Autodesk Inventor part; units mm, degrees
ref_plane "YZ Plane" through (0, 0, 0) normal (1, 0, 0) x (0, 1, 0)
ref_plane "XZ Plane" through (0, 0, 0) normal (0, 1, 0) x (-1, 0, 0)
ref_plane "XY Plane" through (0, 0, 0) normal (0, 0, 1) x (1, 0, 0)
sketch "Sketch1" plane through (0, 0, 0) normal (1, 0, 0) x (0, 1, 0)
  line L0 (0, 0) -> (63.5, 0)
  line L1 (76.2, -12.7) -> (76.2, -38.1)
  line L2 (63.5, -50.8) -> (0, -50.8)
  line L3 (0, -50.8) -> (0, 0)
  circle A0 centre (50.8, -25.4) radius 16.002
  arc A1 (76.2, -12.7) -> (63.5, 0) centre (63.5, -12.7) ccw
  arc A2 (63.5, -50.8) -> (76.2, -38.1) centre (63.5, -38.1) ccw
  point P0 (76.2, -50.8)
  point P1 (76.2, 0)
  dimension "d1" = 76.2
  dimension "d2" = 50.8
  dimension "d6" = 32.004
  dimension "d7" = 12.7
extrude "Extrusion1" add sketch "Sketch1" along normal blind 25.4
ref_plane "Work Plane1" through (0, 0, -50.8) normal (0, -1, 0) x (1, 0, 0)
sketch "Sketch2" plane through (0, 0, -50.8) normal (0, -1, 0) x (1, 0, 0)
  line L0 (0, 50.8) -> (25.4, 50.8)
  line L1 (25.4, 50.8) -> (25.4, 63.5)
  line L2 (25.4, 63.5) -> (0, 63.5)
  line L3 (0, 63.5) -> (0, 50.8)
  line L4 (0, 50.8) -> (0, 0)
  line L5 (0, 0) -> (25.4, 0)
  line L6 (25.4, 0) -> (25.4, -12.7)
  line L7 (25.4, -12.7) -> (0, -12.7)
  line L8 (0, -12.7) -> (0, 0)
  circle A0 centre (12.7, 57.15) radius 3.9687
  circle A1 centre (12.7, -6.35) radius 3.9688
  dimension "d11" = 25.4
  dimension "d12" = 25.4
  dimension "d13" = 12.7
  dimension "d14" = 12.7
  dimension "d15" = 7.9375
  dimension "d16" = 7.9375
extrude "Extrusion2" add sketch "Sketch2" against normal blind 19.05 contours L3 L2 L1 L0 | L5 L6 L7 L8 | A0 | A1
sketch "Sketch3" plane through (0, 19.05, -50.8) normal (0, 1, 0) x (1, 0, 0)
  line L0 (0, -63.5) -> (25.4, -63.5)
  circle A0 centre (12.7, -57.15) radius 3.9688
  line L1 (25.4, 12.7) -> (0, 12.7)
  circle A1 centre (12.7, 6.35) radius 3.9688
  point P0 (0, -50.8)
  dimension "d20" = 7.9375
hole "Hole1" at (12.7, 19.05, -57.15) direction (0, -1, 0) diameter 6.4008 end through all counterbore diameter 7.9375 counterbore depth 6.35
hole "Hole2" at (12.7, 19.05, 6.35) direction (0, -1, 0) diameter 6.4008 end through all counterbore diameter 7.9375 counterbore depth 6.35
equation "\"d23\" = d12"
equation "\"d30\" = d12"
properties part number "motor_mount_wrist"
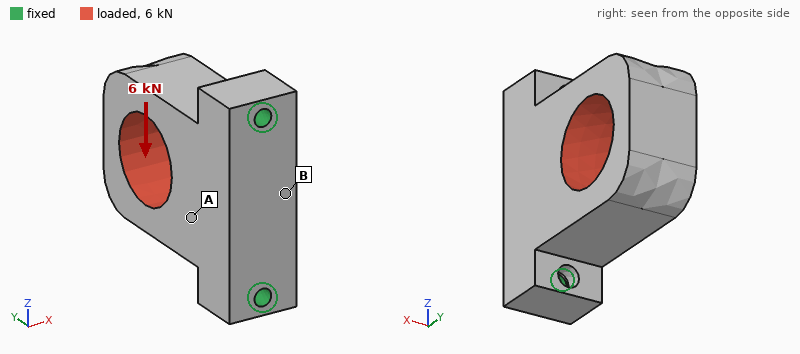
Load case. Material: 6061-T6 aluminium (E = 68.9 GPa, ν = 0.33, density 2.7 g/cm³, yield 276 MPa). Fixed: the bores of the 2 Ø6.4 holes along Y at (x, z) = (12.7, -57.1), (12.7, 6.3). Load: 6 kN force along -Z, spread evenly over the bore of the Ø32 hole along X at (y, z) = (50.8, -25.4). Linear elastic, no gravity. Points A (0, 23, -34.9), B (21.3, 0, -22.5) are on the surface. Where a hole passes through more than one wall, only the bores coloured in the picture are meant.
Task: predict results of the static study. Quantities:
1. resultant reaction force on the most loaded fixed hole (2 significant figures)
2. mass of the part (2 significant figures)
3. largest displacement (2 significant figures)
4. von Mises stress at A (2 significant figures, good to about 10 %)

5.3 kN
230 g
60 µm
13 MPa
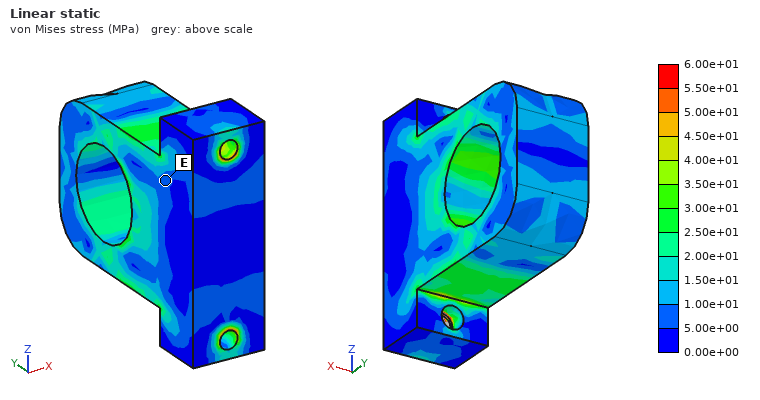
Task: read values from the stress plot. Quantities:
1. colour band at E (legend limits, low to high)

5.00e+00 to 1.00e+01 MPa
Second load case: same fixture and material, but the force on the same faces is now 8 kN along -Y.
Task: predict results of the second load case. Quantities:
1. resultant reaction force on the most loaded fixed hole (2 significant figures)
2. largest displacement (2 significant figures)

4.3 kN
19 µm
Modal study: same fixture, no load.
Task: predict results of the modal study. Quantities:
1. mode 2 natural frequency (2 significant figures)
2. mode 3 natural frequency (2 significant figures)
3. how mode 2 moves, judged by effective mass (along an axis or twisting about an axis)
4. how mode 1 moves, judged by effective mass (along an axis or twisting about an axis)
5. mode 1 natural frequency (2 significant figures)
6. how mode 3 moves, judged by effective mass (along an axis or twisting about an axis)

5300 Hz
7500 Hz
along Z
along X
2400 Hz
twisting about Y
